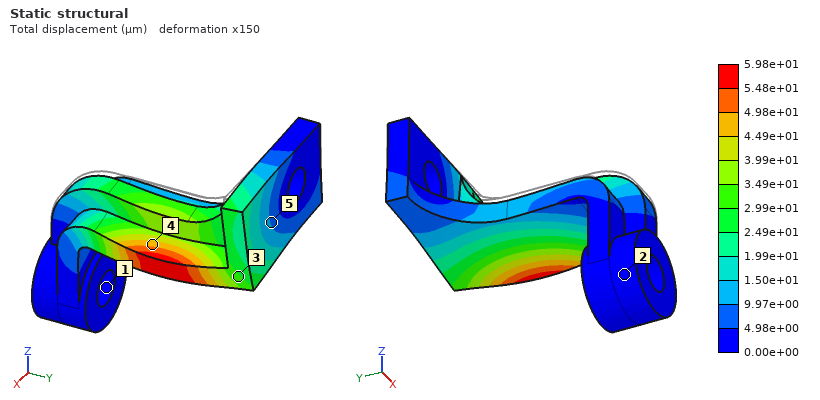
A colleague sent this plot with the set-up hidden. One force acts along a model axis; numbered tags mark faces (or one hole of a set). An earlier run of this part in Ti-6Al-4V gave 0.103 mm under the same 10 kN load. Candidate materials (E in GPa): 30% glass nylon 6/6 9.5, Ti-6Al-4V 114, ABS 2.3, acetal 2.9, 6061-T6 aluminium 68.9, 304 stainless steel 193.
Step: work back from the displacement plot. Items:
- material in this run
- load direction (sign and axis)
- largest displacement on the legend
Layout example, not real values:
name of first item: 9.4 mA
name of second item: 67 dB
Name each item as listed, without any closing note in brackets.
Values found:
material in this run: 304 stainless steel
load direction: -Z
largest displacement on the legend: 5.98e+01 µm
